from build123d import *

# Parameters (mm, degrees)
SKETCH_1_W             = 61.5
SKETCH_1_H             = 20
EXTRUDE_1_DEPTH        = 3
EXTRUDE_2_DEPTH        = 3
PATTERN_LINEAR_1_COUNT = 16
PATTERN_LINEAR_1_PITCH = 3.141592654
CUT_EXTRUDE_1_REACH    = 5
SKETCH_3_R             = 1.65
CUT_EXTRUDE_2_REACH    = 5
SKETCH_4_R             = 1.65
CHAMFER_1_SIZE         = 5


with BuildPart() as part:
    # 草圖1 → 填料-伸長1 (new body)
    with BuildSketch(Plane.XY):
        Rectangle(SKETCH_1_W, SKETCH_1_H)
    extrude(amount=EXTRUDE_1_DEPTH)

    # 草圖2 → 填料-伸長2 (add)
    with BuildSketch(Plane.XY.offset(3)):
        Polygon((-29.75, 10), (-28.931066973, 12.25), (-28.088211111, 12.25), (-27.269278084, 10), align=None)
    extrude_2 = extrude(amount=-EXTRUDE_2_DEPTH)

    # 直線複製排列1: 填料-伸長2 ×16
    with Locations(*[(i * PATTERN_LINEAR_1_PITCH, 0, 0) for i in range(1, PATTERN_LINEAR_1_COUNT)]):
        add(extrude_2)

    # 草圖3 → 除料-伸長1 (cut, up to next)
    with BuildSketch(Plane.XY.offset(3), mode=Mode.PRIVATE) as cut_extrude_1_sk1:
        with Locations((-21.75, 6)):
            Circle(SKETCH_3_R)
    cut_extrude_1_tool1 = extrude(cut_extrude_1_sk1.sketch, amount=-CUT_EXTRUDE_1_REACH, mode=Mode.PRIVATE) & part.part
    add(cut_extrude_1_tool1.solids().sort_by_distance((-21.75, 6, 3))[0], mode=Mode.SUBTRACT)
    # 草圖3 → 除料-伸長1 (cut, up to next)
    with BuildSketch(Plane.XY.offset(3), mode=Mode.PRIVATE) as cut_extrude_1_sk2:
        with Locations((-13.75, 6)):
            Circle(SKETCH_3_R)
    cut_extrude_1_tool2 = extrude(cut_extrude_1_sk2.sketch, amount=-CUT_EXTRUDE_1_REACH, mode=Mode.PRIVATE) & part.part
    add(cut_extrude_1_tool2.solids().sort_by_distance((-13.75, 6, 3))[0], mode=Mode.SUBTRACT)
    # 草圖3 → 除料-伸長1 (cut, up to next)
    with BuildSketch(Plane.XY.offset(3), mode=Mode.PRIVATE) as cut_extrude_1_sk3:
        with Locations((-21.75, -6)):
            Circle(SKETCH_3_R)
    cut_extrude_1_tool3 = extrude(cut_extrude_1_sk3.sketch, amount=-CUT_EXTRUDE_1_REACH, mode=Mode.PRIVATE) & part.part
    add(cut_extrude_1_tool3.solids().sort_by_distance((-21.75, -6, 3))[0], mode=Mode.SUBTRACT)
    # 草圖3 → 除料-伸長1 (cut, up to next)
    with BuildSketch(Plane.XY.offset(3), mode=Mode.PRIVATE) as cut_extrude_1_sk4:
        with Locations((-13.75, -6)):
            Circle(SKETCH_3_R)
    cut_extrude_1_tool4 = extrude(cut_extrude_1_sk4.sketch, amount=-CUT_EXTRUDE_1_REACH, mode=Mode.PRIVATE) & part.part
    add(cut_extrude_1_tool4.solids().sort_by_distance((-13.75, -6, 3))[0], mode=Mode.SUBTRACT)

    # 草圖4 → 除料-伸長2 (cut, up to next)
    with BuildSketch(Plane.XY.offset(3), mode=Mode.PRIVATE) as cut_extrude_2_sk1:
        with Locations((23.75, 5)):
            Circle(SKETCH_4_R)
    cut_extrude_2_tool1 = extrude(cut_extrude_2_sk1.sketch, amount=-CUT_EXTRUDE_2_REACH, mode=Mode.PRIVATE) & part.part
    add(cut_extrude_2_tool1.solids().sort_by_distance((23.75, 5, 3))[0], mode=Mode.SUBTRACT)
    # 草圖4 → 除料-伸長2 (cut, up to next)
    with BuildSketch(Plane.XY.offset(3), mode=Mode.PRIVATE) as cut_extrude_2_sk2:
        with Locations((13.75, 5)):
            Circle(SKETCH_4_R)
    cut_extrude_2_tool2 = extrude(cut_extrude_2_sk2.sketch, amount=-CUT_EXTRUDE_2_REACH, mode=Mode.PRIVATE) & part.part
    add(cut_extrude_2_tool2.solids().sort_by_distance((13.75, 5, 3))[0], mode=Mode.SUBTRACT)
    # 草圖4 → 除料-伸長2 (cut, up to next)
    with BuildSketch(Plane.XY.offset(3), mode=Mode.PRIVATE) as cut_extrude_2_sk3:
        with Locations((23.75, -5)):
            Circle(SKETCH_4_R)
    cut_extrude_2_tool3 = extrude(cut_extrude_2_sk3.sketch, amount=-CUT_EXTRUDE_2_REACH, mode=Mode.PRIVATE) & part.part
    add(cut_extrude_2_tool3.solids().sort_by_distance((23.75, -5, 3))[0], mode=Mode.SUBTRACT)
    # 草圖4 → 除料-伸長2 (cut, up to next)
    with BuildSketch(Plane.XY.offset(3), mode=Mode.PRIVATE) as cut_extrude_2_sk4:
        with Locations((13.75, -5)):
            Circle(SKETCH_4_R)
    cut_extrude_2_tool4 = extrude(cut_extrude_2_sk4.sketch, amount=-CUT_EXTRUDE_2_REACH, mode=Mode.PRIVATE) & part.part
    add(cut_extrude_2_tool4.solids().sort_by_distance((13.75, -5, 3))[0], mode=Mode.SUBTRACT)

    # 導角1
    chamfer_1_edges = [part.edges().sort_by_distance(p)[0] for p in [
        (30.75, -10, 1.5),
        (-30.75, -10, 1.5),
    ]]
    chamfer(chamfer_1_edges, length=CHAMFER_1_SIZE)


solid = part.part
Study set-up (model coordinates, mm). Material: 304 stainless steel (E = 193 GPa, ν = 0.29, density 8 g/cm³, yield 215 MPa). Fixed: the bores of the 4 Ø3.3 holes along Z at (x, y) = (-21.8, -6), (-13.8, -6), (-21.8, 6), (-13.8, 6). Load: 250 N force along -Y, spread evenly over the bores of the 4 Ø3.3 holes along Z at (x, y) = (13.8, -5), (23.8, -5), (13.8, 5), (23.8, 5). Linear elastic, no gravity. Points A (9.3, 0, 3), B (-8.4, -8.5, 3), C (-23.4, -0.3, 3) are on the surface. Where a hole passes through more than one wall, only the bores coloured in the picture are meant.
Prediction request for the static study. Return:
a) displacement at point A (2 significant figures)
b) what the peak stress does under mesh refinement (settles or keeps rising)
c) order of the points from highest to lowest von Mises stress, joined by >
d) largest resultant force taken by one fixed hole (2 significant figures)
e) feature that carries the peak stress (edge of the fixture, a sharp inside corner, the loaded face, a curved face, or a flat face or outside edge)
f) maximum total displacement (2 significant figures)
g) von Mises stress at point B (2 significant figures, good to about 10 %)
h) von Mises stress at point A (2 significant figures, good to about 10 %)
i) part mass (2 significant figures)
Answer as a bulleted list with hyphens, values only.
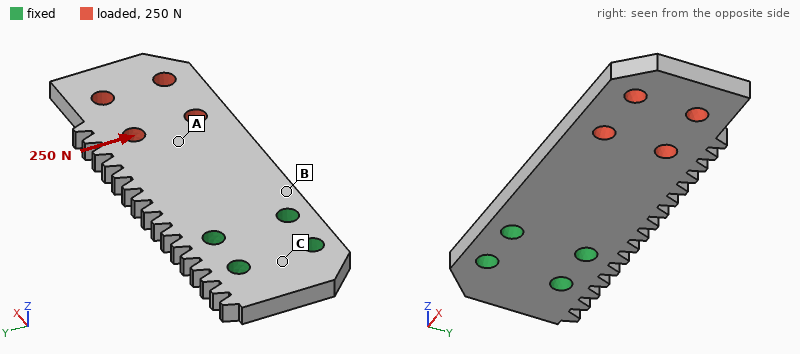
- 5.6 µm
- keeps rising
- B > A > C
- 540 N
- edge of the fixture
- 14 µm
- 27 MPa
- 9.5 MPa
- 29 g
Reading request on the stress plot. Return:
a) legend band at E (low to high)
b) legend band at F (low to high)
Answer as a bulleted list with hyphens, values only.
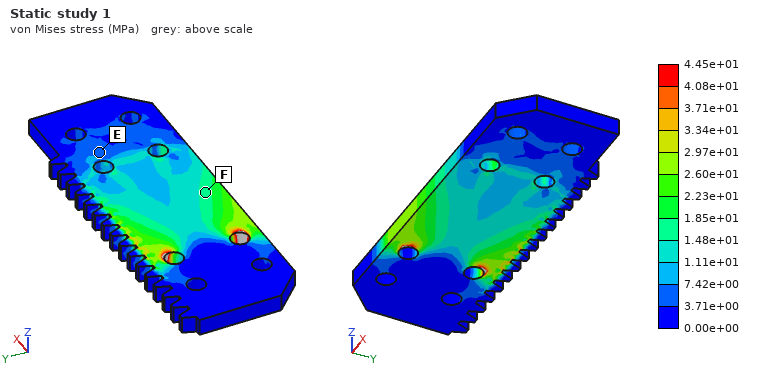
- 3.71e+00 to 7.42e+00 MPa
- 1.48e+01 to 1.85e+01 MPa
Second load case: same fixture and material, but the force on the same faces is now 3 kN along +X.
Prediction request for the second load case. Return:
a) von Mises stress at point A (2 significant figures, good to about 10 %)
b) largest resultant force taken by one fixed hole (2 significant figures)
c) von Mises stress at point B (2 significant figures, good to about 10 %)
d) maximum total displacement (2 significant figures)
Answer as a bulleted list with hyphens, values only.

- 56 MPa
- 1.3 kN
- 51 MPa
- 9.6 µm
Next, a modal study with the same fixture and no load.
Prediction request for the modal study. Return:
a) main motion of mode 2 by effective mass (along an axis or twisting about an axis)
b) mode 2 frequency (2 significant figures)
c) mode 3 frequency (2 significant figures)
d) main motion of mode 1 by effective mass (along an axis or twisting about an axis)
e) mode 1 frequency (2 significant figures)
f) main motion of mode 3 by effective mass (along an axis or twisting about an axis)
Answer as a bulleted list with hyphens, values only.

- twisting about X
- 5600 Hz
- 7300 Hz
- along Z
- 1300 Hz
- along Y
